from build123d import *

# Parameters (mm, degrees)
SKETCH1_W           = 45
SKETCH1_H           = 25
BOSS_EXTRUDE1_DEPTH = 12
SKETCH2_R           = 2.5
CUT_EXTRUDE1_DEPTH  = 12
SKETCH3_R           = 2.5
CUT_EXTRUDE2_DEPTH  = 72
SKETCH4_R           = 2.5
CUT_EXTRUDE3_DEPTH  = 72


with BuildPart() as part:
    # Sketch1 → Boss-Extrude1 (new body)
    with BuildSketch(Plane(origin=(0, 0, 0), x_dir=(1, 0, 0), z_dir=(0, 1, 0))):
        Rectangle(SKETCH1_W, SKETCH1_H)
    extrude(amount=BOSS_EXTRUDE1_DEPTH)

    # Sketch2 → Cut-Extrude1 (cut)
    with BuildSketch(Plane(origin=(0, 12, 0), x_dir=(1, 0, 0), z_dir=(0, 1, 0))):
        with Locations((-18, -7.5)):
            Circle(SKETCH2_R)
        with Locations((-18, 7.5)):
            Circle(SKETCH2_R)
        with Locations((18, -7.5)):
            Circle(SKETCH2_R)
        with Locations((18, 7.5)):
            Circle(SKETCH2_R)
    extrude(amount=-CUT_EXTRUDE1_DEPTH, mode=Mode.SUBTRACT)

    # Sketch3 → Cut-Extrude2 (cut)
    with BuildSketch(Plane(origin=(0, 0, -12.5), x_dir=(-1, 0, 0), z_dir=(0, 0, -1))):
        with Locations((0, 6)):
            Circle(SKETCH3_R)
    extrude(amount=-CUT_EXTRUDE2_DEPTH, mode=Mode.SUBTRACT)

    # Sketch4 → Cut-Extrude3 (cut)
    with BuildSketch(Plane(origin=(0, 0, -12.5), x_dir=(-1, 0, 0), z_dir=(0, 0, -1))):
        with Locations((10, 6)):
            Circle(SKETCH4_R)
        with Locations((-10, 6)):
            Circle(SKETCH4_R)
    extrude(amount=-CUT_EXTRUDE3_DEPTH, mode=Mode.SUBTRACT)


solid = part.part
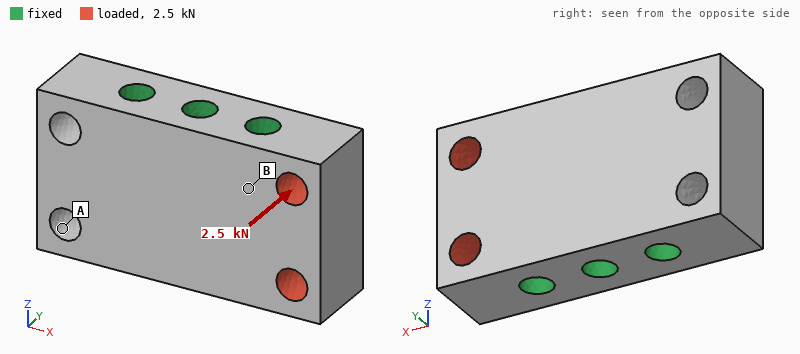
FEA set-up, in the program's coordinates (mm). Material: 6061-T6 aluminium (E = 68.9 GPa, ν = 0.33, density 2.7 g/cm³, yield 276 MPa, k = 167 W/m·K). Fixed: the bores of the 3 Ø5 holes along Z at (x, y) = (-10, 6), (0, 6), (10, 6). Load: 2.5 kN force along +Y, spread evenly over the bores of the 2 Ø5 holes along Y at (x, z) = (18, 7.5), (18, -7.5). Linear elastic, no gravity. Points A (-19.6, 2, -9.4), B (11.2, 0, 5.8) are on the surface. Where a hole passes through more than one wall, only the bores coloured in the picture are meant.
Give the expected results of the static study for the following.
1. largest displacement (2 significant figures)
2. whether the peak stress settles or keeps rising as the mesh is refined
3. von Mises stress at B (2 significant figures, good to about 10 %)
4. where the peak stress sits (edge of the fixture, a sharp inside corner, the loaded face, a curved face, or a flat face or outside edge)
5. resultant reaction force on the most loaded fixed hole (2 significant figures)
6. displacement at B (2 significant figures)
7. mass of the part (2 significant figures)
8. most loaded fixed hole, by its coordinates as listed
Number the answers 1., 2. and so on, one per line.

1. 8.9 µm
2. keeps rising
3. 19 MPa
4. edge of the fixture
5. 3.0 kN
6. 1.6 µm
7. 30 g
8. (10, 6)
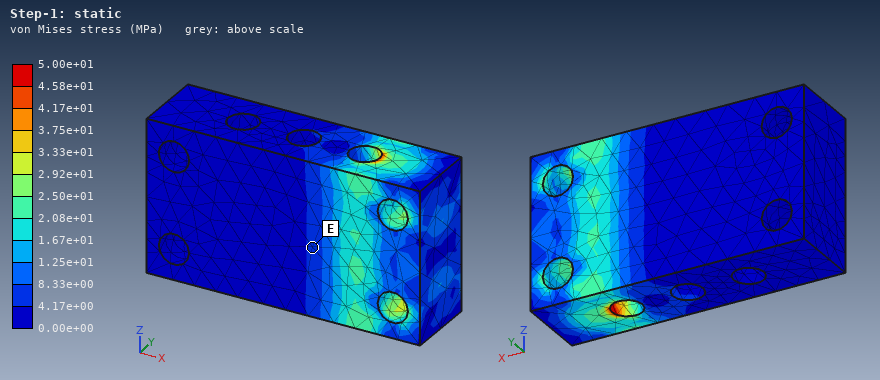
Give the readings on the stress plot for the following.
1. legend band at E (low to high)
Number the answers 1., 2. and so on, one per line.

1. 4.17e+00 to 8.33e+00 MPa
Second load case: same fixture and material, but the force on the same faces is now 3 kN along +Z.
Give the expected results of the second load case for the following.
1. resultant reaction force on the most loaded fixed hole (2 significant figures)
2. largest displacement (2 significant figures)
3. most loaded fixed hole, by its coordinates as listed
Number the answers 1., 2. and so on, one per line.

1. 3.0 kN
2. 5.9 µm
3. (10, 6)
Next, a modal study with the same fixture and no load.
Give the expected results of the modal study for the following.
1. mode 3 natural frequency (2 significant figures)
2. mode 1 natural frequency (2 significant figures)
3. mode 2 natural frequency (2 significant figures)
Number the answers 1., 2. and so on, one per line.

1. 52 kHz
2. 40 kHz
3. 40 kHz
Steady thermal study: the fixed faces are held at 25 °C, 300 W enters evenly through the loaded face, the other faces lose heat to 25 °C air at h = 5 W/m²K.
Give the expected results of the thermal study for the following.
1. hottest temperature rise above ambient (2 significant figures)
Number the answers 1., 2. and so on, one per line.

1. 63 K
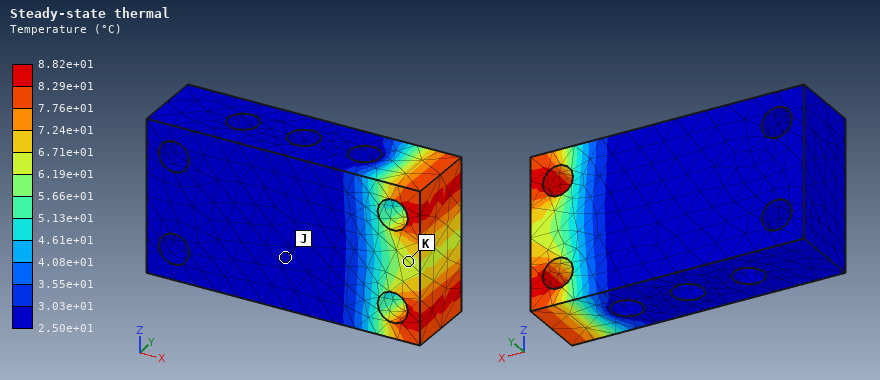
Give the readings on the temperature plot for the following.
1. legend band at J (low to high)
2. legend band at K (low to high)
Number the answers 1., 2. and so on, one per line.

1. 2.50e+01 to 3.03e+01 °C
2. 6.19e+01 to 6.71e+01 °C
